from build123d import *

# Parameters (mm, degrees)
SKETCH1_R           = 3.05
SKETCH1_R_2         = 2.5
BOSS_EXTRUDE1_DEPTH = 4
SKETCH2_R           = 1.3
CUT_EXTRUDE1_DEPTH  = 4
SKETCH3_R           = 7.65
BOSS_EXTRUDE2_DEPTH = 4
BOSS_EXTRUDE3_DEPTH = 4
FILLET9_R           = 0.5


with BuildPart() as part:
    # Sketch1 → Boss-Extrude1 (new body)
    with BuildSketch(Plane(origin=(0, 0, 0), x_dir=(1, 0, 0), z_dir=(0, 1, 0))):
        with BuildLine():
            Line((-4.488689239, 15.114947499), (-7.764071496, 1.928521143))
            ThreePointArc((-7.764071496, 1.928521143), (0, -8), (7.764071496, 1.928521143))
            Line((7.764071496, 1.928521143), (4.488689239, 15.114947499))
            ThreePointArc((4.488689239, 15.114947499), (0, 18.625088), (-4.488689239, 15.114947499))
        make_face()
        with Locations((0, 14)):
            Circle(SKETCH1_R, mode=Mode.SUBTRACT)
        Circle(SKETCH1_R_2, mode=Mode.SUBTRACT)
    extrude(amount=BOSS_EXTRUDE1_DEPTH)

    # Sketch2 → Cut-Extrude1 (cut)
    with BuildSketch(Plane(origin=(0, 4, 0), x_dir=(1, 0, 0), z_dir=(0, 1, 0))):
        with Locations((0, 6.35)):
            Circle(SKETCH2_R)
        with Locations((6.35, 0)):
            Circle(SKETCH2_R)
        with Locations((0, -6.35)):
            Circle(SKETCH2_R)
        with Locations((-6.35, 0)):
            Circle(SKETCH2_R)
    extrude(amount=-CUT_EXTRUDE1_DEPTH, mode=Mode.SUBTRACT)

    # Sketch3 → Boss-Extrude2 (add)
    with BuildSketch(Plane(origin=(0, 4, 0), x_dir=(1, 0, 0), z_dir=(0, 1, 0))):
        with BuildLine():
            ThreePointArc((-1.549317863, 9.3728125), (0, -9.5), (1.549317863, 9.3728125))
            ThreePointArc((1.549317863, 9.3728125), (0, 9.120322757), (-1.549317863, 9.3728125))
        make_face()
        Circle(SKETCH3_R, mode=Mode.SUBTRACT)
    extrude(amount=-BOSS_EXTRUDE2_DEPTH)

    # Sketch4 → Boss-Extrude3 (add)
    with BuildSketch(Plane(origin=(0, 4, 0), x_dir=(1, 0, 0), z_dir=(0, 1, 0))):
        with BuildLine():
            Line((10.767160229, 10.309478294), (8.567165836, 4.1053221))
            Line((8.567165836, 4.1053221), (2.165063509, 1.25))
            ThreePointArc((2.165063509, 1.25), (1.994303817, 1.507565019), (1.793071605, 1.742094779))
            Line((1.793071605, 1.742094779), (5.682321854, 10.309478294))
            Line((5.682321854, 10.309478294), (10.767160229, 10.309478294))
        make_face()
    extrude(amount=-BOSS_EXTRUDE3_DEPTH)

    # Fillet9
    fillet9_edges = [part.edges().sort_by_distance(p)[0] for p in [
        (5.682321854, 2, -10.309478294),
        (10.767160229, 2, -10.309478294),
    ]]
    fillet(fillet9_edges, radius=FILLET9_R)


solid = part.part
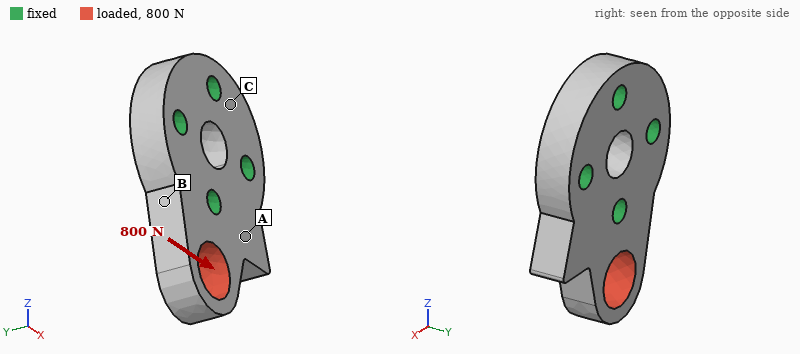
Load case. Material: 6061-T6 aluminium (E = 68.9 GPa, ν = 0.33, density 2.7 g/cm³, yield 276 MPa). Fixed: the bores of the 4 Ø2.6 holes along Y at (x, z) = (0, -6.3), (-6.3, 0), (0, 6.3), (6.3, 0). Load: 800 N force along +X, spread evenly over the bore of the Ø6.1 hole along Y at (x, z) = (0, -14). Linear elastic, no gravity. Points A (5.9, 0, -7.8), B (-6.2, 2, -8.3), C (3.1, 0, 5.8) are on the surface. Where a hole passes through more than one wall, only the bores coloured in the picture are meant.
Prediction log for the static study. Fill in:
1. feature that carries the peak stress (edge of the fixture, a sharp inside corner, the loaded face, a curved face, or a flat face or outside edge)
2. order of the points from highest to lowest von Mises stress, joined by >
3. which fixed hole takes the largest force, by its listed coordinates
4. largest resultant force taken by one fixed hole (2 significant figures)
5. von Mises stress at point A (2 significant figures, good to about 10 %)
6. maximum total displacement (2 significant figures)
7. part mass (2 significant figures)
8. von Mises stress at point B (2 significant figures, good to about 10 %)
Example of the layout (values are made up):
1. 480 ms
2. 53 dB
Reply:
1. a curved face
2. B > A > C
3. (0, -6.3)
4. 790 N
5. 38 MPa
6. 33 µm
7. 3.5 g
8. 67 MPa
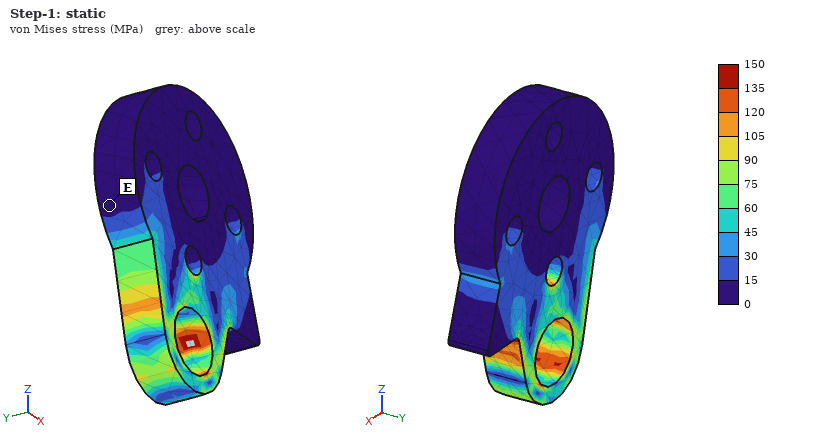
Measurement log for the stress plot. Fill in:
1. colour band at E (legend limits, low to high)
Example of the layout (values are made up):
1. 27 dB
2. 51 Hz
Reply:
1. 0 to 15 MPa
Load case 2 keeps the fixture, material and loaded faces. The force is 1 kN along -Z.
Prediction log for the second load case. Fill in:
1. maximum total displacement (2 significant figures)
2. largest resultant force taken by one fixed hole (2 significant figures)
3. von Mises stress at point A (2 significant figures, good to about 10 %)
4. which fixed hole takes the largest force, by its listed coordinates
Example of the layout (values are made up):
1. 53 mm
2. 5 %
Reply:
1. 10 µm
2. 560 N
3. 17 MPa
4. (0, -6.3)
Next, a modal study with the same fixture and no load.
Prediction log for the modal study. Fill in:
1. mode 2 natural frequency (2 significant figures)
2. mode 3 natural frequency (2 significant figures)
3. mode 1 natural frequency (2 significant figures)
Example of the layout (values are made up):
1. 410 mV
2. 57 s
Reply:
1. 42 kHz
2. 44 kHz
3. 28 kHz
